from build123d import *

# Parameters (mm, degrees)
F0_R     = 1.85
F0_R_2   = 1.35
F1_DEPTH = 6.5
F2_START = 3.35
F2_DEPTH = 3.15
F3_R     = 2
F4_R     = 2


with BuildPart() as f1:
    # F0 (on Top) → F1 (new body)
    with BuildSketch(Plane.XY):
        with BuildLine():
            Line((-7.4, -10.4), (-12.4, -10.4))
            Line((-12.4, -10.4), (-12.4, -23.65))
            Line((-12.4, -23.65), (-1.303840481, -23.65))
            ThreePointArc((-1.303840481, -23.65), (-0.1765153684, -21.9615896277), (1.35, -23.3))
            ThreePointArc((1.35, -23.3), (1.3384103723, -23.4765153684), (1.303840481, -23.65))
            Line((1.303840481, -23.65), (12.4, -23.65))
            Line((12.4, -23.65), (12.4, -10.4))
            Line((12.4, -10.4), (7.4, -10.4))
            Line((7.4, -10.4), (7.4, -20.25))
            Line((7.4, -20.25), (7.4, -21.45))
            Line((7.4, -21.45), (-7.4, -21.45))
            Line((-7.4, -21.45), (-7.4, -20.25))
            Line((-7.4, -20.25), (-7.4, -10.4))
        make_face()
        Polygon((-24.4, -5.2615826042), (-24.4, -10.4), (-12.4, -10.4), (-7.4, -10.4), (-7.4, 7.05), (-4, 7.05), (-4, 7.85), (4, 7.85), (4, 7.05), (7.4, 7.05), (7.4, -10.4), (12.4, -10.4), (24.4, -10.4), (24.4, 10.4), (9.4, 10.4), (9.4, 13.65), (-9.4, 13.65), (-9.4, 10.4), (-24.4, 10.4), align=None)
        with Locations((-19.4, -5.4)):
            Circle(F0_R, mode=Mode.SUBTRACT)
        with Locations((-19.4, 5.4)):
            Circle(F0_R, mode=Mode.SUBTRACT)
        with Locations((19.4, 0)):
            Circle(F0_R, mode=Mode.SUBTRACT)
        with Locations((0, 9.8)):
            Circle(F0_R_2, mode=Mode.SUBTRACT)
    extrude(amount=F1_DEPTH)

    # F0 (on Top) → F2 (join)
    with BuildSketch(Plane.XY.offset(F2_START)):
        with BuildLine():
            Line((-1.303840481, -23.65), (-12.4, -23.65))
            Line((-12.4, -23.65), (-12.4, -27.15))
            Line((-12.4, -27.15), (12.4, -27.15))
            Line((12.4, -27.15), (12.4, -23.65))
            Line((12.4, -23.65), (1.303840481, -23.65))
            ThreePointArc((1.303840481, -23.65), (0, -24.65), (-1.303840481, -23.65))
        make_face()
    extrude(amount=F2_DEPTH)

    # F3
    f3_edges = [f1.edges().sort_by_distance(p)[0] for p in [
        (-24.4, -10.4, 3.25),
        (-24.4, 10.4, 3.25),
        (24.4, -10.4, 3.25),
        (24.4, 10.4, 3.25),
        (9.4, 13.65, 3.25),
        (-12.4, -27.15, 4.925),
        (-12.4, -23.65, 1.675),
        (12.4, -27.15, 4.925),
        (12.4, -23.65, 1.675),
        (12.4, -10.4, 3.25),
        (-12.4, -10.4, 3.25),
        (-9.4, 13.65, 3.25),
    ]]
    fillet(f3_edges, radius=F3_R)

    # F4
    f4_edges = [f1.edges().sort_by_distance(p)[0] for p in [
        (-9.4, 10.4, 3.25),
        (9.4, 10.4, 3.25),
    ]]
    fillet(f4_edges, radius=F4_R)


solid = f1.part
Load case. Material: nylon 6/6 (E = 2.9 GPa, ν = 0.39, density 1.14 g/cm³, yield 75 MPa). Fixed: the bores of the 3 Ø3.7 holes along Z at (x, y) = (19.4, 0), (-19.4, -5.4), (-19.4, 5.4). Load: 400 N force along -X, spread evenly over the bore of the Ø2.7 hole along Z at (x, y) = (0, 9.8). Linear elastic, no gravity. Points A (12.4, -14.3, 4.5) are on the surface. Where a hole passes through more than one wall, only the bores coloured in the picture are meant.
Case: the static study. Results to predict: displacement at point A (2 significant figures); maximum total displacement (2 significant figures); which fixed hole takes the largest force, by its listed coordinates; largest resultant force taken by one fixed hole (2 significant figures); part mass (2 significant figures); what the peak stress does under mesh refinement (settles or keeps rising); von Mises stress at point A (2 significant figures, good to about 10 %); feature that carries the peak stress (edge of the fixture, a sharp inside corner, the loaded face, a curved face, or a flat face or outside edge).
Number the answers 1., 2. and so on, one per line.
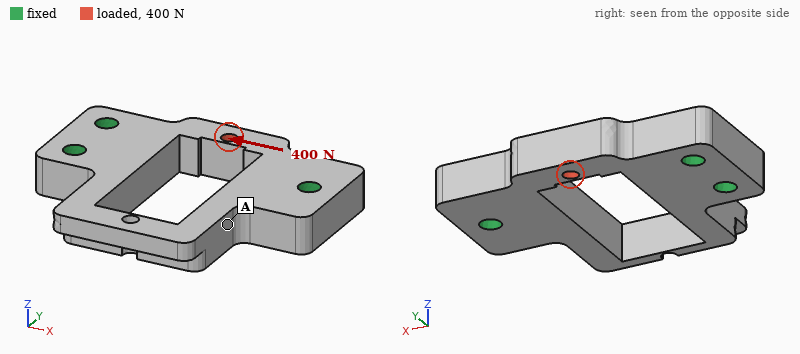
1. 27 µm
2. 61 µm
3. (-19.4, 5.4)
4. 260 N
5. 7.2 g
6. keeps rising
7. 1.8 MPa
8. a sharp inside corner
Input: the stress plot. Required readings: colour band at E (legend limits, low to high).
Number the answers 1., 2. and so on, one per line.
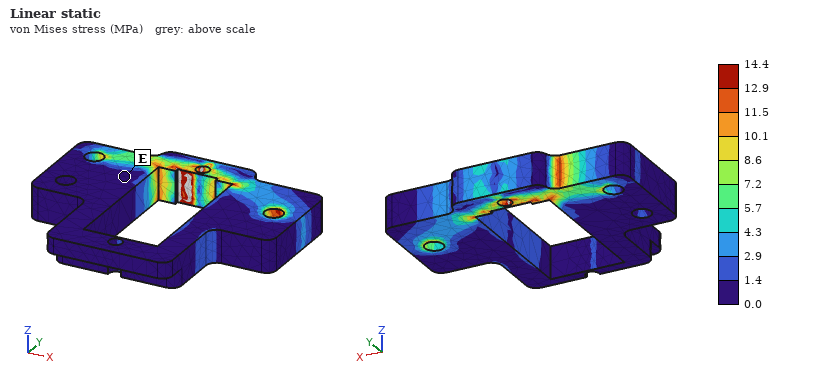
1. 0.0 to 1.4 MPa
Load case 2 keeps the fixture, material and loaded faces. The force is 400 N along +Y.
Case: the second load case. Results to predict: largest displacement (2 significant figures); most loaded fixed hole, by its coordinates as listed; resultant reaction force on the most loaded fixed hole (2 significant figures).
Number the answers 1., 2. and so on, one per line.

1. 0.15 mm
2. (19.4, 0)
3. 280 N
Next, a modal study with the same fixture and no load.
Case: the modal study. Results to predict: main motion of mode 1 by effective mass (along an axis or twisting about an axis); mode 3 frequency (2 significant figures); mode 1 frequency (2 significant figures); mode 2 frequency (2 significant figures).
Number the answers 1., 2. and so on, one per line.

1. along Z
2. 4300 Hz
3. 2400 Hz
4. 4200 Hz
